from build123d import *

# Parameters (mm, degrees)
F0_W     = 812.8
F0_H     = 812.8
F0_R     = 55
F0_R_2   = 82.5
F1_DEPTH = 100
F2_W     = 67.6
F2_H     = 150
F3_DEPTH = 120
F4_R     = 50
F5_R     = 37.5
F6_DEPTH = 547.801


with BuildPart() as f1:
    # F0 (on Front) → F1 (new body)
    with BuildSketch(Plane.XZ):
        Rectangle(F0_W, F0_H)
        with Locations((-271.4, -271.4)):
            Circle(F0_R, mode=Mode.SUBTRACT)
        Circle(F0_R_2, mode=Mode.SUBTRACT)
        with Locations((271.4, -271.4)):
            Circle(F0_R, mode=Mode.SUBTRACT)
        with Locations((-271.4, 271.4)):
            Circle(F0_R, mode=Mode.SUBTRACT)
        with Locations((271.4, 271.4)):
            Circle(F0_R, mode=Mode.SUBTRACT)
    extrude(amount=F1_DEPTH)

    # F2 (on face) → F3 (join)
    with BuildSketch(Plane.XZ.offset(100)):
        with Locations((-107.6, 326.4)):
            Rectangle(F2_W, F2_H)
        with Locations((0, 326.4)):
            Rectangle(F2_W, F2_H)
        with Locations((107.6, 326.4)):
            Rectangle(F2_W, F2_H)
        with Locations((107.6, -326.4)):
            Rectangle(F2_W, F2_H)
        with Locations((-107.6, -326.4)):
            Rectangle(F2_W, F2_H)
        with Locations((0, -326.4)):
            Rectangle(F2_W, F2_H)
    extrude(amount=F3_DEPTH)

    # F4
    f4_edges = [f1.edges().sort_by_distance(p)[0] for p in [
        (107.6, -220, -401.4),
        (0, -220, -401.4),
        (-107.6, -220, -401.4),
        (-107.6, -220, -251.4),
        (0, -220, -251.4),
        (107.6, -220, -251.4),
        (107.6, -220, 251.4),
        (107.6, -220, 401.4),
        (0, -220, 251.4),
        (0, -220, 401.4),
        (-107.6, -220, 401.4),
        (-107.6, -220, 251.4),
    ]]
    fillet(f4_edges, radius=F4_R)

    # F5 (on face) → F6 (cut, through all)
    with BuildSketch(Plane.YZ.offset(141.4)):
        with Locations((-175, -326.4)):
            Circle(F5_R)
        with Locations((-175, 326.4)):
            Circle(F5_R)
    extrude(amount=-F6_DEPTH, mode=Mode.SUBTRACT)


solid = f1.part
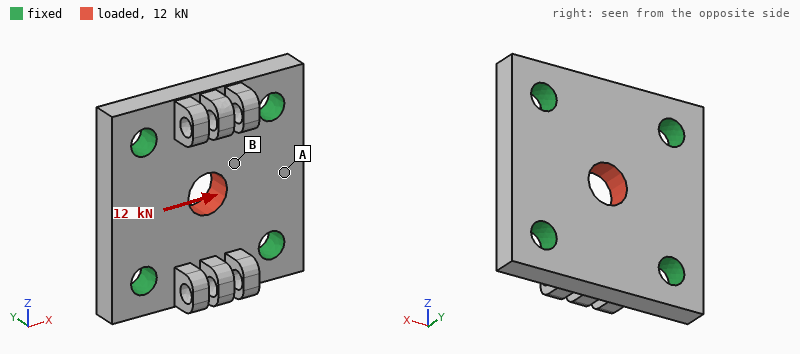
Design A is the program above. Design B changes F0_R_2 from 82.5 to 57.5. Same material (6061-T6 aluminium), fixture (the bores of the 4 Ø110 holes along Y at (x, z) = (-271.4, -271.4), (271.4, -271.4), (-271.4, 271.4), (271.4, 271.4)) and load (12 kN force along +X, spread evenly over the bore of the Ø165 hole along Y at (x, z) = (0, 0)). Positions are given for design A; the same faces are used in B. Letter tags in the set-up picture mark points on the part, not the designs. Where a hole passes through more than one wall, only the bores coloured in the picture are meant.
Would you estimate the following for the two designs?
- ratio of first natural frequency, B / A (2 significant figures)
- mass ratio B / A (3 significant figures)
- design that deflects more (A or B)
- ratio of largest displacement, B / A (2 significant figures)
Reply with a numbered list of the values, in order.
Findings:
1. 0.98
2. 1.02
3. B
4. 1.2
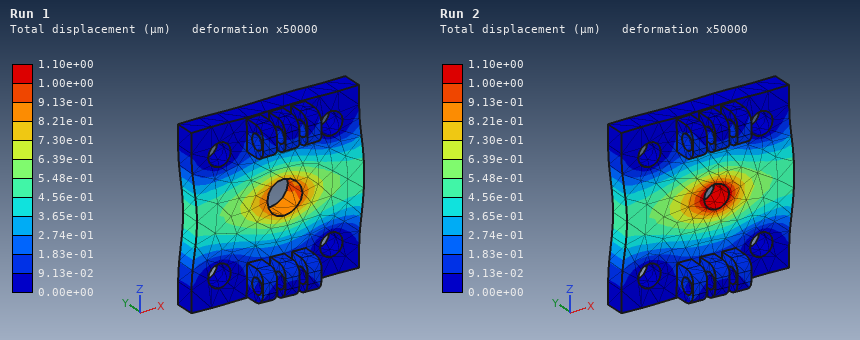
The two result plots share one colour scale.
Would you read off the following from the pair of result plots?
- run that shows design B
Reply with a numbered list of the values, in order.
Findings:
1. Run 2
